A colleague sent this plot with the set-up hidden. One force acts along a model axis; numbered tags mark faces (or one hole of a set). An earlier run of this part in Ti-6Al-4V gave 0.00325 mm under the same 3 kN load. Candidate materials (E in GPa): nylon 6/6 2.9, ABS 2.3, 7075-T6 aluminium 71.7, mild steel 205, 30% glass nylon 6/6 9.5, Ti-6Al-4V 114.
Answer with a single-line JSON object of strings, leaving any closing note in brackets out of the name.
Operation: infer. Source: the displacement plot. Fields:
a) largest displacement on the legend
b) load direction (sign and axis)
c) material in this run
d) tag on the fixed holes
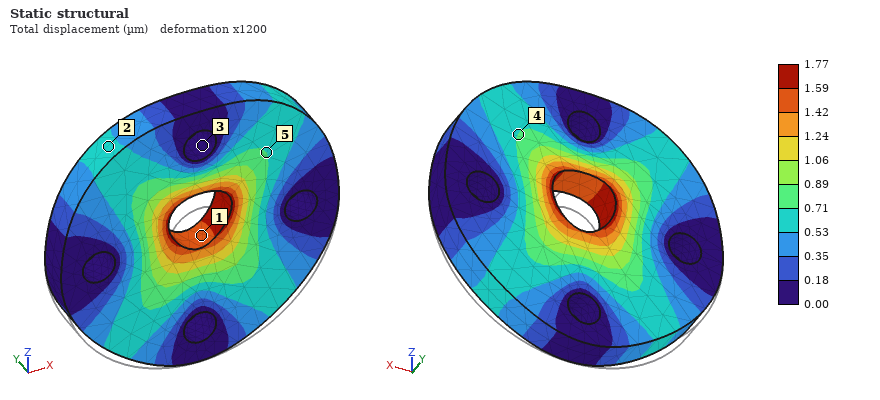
{"largest displacement on the legend": "1.77 µm", "load direction": "+Z", "material in this run": "mild steel", "tag on the fixed holes": "3"}
